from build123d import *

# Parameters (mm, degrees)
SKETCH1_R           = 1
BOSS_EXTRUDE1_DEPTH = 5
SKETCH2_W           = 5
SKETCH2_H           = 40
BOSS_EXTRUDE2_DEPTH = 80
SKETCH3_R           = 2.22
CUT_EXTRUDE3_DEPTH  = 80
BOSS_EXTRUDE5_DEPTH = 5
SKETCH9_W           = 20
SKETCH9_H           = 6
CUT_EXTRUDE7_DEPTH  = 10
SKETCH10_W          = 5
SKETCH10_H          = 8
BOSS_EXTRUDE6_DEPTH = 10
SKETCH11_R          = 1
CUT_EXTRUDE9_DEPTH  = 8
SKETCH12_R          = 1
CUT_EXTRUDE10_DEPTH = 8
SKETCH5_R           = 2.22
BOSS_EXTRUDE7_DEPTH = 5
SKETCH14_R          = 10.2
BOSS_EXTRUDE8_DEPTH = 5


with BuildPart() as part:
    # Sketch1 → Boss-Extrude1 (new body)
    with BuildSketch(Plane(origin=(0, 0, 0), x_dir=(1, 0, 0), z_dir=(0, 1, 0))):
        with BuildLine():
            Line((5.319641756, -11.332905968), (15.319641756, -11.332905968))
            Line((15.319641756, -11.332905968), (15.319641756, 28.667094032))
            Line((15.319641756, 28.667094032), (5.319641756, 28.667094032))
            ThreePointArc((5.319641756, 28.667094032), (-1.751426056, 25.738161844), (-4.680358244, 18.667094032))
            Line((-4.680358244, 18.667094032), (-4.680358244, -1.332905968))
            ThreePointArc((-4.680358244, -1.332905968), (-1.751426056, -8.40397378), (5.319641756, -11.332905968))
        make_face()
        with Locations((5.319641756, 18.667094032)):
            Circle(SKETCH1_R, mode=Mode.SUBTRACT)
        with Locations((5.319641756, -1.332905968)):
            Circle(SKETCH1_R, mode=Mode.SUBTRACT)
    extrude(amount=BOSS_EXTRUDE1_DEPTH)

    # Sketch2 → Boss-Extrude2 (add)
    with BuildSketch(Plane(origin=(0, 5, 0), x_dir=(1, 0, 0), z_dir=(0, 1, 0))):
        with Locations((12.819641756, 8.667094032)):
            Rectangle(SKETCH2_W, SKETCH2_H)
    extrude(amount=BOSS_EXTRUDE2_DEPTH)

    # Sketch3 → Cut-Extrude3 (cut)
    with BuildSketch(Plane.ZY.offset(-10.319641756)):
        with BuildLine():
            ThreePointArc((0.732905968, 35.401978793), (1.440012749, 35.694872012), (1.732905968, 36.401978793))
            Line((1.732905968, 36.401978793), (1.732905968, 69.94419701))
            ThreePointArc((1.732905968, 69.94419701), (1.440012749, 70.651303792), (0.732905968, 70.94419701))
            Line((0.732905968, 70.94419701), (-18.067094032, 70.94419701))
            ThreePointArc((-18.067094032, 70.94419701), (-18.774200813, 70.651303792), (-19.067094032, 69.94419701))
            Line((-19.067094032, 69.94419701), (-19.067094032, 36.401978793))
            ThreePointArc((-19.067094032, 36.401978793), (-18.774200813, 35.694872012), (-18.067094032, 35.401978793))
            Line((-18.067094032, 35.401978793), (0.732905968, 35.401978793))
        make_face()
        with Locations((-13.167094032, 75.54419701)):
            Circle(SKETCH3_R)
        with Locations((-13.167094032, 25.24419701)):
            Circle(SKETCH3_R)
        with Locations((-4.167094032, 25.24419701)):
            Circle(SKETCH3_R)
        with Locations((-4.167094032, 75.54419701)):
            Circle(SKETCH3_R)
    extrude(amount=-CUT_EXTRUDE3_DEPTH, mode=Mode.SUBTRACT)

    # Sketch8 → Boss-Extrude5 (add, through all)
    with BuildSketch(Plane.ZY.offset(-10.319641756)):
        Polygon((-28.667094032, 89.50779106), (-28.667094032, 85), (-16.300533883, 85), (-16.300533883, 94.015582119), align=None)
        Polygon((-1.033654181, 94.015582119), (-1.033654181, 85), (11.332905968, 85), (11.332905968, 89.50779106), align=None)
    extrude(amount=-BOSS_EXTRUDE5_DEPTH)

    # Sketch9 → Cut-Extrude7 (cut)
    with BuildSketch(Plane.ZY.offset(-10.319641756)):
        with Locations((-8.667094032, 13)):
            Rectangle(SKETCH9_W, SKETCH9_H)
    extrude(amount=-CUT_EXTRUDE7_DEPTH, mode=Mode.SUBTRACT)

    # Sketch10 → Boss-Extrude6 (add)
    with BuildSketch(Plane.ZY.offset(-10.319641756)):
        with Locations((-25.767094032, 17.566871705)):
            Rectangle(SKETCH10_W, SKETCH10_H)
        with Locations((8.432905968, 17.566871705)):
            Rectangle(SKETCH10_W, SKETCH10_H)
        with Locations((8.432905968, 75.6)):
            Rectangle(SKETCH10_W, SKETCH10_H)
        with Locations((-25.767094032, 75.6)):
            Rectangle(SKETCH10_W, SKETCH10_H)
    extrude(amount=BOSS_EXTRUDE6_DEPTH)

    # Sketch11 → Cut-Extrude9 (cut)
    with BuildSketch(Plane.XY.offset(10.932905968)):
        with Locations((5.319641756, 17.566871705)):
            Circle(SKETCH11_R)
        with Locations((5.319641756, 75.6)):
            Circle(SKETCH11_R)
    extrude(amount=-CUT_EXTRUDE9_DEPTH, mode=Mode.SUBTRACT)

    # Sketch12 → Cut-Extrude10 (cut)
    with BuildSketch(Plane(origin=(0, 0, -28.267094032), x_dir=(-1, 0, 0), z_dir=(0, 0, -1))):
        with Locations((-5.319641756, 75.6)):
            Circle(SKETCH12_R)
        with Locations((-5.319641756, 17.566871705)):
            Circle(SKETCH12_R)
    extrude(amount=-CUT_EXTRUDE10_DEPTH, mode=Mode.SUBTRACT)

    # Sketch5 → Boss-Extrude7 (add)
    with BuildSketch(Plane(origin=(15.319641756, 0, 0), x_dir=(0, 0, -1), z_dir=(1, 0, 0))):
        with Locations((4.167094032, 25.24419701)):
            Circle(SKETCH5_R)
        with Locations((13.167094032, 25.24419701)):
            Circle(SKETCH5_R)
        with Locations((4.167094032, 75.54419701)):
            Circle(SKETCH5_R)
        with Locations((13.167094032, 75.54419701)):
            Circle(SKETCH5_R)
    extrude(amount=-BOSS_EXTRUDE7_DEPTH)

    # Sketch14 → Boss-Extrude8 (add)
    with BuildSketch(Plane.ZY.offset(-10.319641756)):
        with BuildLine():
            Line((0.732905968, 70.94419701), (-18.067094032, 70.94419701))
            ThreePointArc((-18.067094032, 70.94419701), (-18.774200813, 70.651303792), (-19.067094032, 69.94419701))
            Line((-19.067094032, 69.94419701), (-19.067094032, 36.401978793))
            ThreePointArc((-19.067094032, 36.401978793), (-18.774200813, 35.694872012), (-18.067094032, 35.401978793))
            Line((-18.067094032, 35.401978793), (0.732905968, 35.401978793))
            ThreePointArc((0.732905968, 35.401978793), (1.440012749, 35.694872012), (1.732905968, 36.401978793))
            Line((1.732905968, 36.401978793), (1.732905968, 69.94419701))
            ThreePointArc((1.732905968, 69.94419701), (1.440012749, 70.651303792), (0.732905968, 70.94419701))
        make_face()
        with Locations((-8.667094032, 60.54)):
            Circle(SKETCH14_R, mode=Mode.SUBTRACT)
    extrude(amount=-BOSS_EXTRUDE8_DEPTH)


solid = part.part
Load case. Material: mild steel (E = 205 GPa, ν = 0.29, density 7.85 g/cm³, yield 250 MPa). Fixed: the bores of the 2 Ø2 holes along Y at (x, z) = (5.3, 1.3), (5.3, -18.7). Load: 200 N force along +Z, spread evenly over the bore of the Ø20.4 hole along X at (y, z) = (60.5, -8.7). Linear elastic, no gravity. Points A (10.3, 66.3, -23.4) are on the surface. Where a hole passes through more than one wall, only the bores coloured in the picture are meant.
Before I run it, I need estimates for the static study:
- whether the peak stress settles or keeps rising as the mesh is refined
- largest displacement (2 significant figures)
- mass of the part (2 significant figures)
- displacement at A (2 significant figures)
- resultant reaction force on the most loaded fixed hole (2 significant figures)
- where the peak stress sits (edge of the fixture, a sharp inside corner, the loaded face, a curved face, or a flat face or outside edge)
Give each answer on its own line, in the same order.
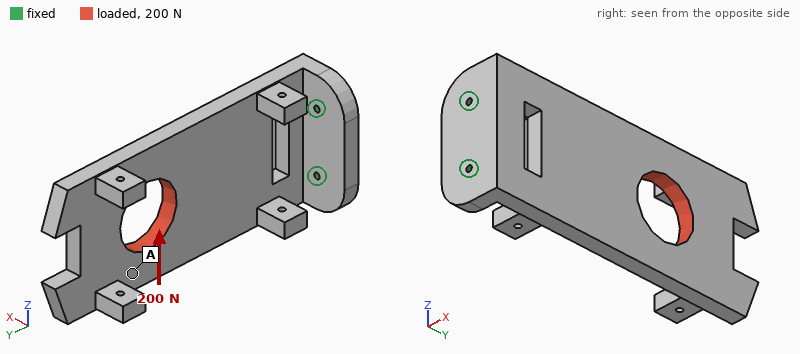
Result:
keeps rising
28 µm
160 g
21 µm
500 N
edge of the fixture
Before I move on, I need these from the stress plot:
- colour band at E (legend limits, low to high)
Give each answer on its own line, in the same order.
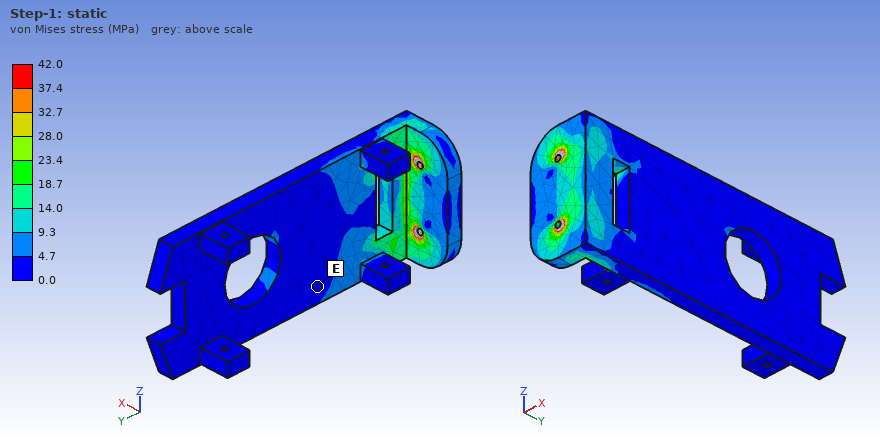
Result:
0.0 to 4.7 MPa
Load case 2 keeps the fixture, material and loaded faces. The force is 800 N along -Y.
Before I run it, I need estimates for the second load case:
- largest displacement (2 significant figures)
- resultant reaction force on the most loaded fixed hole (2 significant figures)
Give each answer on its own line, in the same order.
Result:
48 µm
400 N
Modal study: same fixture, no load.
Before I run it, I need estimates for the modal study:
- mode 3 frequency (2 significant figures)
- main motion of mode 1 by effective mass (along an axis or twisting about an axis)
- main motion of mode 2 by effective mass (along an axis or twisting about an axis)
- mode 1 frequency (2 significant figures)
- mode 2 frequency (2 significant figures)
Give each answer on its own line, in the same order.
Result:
2000 Hz
along X
along Z
400 Hz
1600 Hz
